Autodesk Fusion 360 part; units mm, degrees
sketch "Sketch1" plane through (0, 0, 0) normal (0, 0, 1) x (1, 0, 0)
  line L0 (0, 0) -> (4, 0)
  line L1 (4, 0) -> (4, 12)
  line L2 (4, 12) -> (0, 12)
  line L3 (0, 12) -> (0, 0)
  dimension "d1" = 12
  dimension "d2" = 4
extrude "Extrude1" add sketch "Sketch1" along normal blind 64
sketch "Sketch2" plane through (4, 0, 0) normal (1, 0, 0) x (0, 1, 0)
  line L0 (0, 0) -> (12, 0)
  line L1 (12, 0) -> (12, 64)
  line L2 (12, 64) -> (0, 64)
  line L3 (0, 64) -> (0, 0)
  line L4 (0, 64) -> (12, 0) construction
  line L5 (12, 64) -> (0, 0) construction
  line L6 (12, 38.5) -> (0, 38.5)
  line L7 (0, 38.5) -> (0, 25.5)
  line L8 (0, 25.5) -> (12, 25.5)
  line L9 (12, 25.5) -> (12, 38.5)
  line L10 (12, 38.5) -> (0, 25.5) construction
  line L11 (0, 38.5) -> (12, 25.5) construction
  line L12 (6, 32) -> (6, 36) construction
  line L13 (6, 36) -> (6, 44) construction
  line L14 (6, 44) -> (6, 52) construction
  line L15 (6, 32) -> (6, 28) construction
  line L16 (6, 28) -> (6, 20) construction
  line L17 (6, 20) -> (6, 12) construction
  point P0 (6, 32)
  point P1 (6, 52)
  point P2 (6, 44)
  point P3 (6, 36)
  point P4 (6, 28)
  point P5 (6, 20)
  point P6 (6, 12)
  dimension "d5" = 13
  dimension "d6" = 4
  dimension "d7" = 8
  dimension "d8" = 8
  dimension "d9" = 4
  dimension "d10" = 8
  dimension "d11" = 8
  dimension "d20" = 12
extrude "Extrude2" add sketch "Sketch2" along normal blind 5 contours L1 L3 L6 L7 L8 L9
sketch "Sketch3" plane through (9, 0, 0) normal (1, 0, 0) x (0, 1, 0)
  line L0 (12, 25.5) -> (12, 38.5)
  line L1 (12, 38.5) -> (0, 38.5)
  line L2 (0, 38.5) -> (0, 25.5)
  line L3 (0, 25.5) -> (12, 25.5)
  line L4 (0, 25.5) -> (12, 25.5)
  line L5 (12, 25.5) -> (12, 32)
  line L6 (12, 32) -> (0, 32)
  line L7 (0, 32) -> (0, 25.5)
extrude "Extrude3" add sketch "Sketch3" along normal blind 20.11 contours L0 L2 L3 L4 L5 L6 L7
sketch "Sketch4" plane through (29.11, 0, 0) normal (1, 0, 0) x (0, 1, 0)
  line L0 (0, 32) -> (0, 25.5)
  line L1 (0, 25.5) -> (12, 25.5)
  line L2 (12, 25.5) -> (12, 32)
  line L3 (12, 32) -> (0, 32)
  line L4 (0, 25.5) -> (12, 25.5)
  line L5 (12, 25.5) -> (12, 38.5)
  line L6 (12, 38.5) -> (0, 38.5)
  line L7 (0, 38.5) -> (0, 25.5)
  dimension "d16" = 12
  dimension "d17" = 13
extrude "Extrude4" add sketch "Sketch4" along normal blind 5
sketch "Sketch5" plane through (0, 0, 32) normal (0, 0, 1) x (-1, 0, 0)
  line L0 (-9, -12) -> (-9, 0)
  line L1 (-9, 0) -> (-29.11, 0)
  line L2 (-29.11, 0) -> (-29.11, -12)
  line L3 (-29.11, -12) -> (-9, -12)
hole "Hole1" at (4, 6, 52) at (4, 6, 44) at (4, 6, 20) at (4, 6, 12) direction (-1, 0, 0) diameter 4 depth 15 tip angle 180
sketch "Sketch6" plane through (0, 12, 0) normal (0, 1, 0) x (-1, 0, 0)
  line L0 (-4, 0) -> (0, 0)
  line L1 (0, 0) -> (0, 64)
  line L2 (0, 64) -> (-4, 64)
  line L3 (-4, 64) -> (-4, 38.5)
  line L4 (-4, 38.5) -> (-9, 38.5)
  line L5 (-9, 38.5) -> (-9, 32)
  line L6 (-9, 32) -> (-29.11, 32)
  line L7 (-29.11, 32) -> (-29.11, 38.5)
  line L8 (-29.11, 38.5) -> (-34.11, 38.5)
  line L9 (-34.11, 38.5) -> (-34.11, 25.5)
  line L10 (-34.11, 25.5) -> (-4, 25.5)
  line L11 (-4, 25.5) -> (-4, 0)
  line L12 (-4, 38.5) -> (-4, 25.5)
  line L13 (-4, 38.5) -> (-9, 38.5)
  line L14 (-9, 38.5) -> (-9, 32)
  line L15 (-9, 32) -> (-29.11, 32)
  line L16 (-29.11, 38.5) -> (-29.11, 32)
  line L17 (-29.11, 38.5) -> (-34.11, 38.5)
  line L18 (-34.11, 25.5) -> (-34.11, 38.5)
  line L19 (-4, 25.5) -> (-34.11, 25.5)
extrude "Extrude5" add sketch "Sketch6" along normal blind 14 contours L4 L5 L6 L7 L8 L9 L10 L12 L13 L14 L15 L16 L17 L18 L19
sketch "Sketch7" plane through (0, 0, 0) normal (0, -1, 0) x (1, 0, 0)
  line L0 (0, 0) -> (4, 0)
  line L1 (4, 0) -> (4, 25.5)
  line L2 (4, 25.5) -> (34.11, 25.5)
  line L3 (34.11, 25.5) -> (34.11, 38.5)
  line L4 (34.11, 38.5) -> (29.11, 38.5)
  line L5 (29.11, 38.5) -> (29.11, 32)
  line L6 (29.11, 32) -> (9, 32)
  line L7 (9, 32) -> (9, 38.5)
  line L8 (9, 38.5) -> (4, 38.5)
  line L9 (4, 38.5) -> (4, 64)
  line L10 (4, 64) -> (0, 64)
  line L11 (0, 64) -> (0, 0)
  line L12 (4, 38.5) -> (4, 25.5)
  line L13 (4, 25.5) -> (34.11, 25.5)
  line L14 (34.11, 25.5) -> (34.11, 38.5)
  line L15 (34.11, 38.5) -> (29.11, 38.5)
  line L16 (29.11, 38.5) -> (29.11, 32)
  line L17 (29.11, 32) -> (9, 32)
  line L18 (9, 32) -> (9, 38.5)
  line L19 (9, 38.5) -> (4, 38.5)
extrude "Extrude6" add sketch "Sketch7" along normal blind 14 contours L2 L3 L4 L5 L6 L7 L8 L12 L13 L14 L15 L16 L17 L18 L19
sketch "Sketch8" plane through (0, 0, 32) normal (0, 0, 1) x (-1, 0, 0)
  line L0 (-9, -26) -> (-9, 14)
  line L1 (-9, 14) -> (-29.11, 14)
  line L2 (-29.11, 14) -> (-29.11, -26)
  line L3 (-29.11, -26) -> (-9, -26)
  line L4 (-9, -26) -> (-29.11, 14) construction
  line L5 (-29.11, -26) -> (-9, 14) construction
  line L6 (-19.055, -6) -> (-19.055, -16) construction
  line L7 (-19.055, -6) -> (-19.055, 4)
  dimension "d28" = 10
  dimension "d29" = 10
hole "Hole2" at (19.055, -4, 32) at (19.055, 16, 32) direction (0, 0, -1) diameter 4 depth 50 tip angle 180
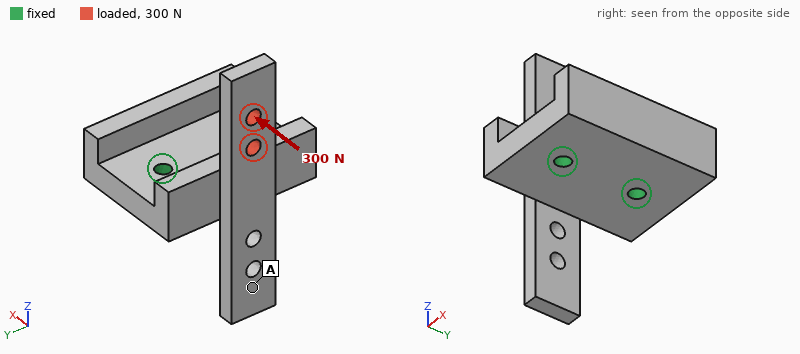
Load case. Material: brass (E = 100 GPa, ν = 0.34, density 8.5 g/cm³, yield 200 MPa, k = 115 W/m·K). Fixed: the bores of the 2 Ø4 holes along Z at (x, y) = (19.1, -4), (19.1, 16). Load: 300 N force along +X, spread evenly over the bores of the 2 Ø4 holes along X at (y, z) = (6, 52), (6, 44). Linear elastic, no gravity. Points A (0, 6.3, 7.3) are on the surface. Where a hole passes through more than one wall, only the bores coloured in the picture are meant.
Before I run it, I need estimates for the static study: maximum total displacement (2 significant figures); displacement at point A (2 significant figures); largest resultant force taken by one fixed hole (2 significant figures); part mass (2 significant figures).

0.14 mm
0.027 mm
160 N
110 g
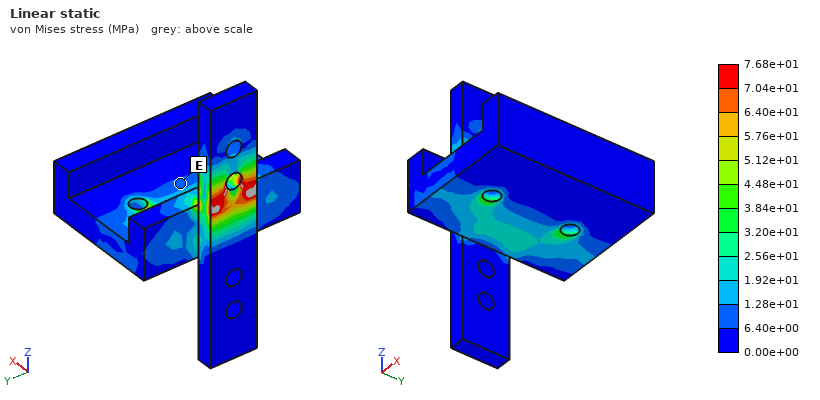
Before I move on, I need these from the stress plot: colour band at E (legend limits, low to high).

6.40e+00 to 1.28e+01 MPa
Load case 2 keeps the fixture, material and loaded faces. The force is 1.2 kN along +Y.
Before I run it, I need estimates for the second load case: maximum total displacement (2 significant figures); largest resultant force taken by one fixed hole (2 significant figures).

0.11 mm
1.4 kN
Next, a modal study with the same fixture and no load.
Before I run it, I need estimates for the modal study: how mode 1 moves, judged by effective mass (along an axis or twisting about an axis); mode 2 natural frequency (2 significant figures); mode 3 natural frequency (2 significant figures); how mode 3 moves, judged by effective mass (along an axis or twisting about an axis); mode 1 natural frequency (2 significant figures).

twisting about Y
2700 Hz
4800 Hz
twisting about X
2200 Hz
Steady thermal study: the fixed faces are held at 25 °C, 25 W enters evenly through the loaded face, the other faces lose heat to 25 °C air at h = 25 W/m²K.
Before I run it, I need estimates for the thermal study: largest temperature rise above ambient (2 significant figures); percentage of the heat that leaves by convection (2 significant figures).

83 K
9.3 %
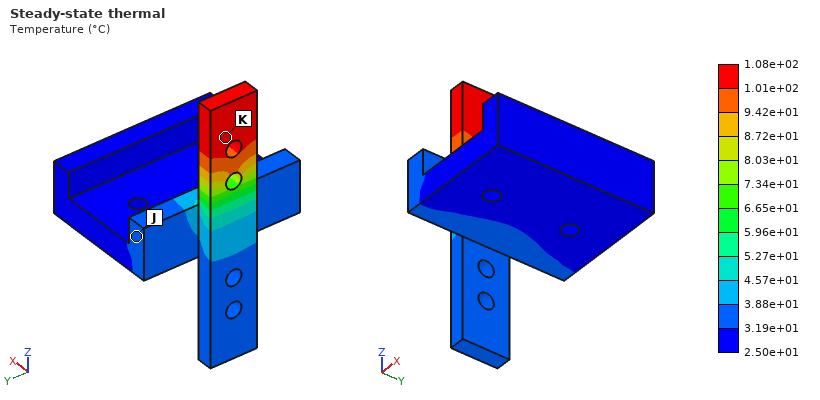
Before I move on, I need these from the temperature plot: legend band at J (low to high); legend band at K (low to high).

3.19e+01 to 3.88e+01 °C
1.01e+02 to 1.08e+02 °C
